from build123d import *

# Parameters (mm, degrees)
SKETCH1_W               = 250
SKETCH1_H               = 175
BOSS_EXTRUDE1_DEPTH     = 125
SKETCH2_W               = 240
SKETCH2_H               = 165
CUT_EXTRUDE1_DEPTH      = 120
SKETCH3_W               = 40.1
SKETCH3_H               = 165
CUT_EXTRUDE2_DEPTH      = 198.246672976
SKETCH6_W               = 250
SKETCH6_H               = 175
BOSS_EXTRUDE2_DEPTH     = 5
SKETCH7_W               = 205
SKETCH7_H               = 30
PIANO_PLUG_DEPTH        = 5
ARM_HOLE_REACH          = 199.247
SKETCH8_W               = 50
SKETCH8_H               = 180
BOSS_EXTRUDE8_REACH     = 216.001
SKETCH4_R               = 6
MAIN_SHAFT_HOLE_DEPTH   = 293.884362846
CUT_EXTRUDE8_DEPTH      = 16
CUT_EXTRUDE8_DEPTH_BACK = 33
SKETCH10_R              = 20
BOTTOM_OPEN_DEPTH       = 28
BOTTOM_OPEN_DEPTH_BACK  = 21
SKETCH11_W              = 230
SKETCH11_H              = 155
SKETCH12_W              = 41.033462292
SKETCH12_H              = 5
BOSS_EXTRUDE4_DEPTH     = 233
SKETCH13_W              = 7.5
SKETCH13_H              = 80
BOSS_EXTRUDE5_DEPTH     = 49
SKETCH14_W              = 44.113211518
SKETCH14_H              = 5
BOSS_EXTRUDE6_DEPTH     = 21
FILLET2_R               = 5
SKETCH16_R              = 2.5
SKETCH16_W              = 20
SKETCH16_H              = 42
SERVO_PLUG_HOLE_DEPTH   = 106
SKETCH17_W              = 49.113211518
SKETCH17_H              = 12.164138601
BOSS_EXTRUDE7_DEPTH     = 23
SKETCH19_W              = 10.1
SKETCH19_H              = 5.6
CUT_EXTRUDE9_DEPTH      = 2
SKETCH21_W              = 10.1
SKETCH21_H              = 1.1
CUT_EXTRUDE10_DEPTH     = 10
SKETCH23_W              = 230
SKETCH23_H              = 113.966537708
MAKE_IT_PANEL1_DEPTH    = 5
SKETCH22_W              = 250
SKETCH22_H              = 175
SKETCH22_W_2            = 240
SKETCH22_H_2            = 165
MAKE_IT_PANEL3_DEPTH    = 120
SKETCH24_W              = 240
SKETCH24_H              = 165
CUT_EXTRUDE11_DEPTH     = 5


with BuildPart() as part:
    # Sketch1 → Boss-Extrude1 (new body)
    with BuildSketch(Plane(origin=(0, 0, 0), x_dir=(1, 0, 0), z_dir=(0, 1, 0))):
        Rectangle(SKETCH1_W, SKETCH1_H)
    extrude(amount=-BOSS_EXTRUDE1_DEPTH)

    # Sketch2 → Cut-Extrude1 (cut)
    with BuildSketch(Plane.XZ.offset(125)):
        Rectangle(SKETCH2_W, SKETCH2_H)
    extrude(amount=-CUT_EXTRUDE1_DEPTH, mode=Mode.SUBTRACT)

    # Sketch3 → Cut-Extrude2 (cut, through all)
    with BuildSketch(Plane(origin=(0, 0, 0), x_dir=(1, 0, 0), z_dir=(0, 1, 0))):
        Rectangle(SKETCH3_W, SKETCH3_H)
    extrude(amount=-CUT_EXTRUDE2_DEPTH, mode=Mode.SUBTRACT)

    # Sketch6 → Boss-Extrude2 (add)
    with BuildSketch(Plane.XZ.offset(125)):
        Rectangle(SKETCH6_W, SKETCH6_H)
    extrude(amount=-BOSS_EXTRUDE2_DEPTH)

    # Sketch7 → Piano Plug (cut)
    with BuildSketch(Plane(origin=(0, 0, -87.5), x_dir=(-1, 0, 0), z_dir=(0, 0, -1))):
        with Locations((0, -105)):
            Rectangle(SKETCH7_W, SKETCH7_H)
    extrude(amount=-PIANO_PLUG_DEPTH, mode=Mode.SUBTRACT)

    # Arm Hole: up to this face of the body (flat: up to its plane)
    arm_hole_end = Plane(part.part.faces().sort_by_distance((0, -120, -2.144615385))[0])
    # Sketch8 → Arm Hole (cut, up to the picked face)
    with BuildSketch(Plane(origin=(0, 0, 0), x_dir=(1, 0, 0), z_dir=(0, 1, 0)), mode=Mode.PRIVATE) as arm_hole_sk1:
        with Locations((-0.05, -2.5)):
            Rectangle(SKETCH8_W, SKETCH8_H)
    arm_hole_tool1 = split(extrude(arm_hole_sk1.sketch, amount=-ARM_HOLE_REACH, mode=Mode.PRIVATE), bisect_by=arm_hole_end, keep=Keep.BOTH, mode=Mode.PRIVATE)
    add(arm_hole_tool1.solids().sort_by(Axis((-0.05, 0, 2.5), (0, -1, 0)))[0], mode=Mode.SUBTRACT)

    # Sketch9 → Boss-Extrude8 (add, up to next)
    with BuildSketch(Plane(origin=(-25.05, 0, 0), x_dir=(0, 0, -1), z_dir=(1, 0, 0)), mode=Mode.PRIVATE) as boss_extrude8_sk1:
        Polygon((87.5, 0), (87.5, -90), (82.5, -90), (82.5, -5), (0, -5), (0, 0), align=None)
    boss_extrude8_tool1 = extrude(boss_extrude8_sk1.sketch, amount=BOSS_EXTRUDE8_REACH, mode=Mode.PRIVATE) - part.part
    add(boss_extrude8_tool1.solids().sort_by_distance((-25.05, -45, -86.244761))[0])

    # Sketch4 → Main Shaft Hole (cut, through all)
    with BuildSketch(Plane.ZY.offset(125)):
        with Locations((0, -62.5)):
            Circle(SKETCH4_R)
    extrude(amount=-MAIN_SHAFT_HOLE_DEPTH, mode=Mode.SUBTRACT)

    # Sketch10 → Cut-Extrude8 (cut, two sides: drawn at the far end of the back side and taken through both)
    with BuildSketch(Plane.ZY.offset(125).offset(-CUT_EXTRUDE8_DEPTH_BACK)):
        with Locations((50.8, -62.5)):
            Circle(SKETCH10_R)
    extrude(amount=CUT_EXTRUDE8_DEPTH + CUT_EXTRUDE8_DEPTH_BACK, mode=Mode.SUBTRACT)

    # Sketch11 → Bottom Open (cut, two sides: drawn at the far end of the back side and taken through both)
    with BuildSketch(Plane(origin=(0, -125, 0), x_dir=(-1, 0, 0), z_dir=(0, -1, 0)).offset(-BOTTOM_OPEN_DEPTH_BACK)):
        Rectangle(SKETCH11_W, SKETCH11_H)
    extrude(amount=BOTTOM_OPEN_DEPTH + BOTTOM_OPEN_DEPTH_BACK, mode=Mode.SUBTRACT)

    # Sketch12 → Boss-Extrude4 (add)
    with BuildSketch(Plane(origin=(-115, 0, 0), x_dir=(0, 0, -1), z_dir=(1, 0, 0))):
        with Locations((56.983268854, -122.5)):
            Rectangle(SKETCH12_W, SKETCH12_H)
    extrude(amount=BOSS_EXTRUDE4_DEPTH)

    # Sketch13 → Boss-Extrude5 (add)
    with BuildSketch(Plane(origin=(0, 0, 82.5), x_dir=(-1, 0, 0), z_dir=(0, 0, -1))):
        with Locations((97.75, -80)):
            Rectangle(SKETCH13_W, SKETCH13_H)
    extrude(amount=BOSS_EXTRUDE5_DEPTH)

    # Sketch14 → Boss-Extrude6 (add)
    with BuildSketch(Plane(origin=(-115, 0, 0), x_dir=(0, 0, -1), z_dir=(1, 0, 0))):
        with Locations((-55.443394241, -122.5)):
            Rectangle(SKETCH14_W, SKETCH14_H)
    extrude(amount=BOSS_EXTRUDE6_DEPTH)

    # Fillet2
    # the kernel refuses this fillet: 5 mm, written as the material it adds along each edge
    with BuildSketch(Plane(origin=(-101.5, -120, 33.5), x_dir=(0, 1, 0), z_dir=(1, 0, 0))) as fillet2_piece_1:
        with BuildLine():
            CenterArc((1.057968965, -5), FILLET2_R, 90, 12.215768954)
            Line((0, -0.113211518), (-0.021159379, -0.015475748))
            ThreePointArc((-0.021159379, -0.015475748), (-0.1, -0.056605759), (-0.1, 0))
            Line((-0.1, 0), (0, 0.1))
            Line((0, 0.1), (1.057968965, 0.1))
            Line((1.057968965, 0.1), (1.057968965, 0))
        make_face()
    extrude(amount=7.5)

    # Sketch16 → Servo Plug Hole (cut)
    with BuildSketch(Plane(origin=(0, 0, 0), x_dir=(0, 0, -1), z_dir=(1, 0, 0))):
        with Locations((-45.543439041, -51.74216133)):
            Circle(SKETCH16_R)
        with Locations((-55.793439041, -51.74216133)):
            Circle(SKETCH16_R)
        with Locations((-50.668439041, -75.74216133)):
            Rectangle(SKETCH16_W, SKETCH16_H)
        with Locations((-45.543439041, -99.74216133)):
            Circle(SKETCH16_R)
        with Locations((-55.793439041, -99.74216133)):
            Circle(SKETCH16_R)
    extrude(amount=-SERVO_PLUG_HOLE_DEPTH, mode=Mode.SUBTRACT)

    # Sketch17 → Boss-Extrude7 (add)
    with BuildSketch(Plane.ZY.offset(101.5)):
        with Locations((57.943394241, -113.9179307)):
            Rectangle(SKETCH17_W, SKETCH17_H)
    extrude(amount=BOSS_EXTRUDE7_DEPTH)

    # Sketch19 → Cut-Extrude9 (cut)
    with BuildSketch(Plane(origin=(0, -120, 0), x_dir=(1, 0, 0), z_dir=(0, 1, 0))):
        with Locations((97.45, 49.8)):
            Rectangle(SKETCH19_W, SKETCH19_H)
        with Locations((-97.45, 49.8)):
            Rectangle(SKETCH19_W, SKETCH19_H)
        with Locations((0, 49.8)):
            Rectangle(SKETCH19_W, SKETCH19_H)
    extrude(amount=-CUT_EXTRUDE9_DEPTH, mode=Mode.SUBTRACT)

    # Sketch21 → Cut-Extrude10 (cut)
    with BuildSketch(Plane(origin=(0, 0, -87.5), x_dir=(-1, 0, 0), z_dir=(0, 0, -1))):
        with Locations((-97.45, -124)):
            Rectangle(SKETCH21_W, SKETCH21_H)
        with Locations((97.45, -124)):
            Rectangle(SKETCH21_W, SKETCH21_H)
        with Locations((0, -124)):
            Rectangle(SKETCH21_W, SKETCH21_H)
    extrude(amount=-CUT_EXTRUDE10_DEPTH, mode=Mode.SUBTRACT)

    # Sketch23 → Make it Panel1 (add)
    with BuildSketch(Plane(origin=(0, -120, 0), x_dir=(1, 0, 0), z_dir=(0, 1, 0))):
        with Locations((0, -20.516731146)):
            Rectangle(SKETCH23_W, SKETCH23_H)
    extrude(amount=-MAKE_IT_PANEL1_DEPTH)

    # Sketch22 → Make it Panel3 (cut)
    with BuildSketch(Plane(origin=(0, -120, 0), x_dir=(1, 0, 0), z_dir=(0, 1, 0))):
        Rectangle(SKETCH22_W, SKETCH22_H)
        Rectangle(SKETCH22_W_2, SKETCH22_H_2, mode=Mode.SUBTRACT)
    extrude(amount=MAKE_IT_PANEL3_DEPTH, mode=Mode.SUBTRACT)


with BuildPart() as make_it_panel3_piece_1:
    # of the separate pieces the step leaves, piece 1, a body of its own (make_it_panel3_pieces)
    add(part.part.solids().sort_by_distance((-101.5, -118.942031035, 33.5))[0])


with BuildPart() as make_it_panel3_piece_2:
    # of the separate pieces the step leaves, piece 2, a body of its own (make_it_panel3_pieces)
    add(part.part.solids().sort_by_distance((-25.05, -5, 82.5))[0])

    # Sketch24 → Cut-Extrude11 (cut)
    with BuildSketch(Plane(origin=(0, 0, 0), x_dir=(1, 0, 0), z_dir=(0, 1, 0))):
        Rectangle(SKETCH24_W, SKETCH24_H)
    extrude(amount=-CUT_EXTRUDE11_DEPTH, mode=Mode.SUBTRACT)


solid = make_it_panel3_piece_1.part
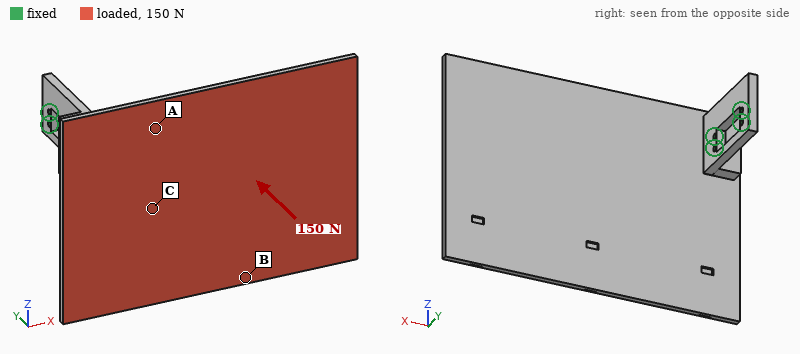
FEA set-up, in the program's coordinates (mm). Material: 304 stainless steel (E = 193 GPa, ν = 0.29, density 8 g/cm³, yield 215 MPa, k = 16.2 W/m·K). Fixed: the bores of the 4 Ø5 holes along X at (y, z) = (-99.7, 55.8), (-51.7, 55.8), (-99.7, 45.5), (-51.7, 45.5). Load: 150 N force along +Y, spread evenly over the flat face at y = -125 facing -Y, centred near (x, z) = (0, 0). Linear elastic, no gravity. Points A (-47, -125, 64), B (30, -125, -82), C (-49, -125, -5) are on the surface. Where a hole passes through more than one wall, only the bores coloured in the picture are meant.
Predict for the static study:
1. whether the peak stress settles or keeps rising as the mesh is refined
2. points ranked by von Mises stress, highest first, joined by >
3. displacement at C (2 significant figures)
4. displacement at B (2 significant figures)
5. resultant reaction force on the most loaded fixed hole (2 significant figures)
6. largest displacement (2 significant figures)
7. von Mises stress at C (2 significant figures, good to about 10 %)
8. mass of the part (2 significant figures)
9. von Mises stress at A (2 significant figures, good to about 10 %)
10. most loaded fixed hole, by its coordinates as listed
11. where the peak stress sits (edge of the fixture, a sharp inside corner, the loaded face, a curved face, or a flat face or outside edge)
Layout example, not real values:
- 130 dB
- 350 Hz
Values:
- keeps rising
- A > C > B
- 0.16 mm
- 0.58 mm
- 360 N
- 1.0 mm
- 11 MPa
- 2.0 kg
- 18 MPa
- (-99.7, 45.5)
- a sharp inside corner
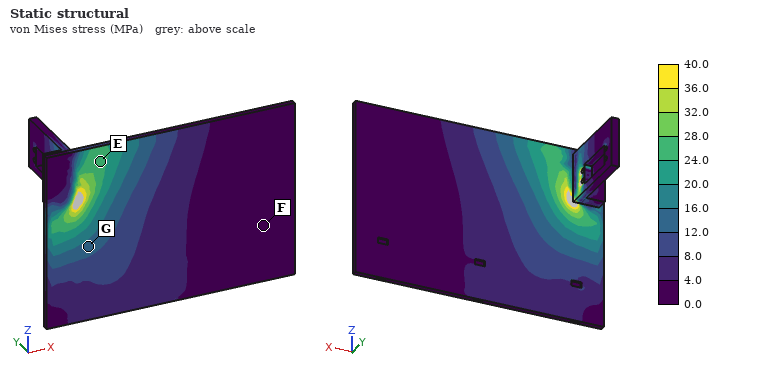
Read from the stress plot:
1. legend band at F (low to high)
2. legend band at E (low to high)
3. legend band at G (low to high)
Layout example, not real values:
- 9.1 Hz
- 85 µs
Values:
- 0.0 to 4.0 MPa
- 24.0 to 28.0 MPa
- 12.0 to 16.0 MPa
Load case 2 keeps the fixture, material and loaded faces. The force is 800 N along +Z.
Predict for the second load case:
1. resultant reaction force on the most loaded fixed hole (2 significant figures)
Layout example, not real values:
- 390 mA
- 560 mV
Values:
- 3.5 kN
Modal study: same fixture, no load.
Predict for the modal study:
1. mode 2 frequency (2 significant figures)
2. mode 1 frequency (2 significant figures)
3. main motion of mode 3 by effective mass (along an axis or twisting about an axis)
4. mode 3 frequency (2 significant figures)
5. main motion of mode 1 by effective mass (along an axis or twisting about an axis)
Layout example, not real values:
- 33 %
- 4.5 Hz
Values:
- 160 Hz
- 60 Hz
- along Z
- 200 Hz
- along Y
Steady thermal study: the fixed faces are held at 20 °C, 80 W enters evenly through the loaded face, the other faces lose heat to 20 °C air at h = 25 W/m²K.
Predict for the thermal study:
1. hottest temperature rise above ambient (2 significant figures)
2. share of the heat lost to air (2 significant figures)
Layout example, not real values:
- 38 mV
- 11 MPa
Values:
- 67 K
- 91 %
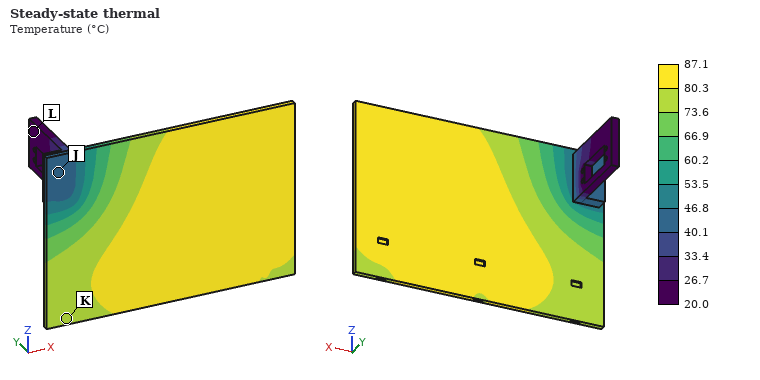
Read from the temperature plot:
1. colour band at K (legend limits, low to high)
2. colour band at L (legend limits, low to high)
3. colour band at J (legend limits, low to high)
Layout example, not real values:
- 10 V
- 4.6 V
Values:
- 73.6 to 80.3 °C
- 20.0 to 26.7 °C
- 40.1 to 46.8 °C
